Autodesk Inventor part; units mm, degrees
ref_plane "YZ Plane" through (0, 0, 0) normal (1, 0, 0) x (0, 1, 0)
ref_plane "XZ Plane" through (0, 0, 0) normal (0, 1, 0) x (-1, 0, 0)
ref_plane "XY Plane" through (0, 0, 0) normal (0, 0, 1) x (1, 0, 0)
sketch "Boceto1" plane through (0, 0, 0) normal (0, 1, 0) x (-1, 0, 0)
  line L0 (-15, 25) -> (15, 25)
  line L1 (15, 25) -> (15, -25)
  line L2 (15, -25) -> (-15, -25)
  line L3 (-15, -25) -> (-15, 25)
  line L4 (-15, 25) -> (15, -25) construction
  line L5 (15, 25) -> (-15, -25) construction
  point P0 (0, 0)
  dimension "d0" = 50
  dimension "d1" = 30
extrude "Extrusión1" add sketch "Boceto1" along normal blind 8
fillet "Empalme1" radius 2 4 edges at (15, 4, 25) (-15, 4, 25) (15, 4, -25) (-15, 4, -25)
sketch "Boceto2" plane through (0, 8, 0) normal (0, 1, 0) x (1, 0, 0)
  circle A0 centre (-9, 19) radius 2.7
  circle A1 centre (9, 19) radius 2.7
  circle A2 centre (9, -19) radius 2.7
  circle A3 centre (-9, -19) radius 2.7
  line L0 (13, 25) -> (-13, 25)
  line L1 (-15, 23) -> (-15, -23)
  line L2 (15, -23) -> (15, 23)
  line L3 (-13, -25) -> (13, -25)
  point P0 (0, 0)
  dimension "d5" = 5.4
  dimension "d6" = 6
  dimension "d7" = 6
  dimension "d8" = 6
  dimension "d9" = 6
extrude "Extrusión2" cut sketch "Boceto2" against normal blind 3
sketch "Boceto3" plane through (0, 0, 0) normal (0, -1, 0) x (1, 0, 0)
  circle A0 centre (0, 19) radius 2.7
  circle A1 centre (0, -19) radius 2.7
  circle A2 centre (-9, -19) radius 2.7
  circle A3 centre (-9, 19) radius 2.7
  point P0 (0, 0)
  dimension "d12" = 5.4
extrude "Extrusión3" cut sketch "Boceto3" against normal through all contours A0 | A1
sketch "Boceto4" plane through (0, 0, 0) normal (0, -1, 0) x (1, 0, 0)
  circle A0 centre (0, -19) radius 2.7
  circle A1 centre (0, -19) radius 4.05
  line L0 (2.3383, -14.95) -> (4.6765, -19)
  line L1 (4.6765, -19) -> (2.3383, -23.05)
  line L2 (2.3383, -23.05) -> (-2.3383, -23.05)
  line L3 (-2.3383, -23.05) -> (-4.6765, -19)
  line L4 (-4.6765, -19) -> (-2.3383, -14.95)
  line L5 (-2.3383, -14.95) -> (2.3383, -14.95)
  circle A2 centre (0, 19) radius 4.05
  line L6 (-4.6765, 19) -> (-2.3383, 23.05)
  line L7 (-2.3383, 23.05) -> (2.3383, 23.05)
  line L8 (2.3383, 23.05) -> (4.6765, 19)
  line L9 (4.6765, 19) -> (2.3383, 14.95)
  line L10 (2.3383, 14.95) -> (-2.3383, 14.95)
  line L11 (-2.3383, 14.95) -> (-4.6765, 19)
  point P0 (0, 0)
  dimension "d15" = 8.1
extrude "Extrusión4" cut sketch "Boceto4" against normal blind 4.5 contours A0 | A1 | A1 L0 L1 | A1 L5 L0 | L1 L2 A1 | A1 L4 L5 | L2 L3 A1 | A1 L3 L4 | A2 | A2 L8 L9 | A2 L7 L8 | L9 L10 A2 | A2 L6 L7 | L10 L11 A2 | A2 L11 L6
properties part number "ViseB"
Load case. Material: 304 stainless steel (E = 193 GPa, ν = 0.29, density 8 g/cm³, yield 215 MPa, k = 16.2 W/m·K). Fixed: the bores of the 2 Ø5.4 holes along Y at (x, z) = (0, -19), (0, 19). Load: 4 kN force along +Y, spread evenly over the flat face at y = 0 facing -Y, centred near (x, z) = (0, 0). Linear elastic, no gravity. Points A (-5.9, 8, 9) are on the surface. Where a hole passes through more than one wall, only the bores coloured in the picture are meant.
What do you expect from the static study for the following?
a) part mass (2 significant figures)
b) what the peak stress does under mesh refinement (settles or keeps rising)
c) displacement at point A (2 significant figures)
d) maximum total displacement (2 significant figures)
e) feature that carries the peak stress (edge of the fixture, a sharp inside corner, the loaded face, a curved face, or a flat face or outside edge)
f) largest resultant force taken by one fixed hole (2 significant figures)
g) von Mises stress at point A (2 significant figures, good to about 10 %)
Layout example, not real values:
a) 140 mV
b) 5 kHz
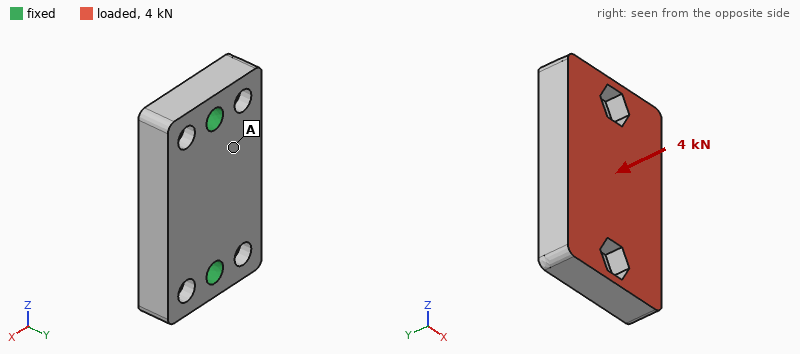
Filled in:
a) 88 g
b) keeps rising
c) 5.1 µm
d) 8.4 µm
e) edge of the fixture
f) 2.2 kN
g) 17 MPa
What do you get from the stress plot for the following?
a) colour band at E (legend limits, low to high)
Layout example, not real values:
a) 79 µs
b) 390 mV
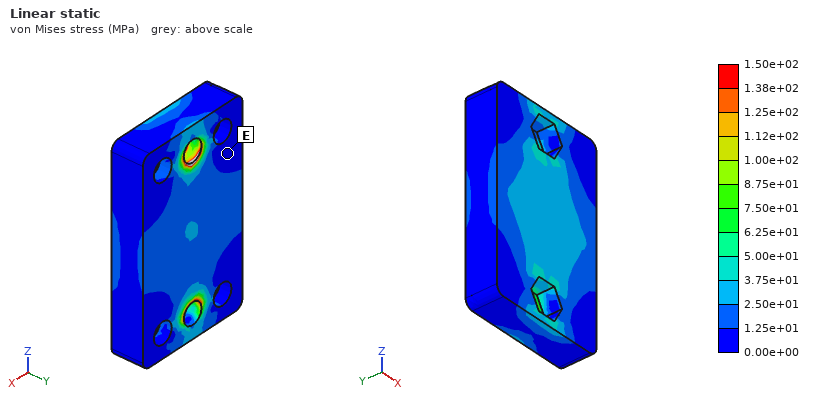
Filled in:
a) 0.00e+00 to 1.25e+01 MPa
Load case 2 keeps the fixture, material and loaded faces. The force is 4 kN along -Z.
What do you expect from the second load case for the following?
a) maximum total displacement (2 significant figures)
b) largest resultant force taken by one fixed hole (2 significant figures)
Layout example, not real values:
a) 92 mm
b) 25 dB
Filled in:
a) 3.0 µm
b) 2.1 kN
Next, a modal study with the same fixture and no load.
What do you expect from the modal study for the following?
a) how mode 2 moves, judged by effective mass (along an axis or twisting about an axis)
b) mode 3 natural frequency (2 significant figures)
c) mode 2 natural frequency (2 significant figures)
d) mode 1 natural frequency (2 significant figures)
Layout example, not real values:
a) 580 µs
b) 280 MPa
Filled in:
a) along Y
b) 19 kHz
c) 14 kHz
d) 8600 Hz
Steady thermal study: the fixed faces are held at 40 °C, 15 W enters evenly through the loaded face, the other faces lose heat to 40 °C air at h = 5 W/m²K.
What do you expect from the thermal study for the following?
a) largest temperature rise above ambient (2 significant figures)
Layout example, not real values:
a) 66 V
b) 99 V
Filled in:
a) 35 K
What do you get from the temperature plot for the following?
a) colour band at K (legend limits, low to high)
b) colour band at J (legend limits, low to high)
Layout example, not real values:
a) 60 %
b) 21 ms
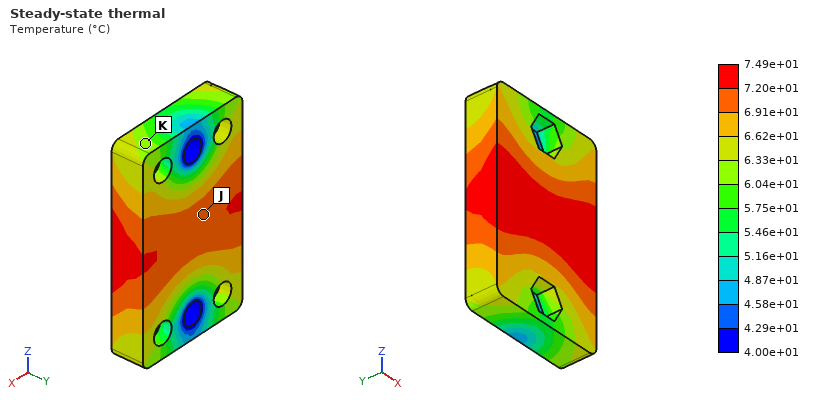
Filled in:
a) 6.04e+01 to 6.33e+01 °C
b) 6.91e+01 to 7.20e+01 °C
